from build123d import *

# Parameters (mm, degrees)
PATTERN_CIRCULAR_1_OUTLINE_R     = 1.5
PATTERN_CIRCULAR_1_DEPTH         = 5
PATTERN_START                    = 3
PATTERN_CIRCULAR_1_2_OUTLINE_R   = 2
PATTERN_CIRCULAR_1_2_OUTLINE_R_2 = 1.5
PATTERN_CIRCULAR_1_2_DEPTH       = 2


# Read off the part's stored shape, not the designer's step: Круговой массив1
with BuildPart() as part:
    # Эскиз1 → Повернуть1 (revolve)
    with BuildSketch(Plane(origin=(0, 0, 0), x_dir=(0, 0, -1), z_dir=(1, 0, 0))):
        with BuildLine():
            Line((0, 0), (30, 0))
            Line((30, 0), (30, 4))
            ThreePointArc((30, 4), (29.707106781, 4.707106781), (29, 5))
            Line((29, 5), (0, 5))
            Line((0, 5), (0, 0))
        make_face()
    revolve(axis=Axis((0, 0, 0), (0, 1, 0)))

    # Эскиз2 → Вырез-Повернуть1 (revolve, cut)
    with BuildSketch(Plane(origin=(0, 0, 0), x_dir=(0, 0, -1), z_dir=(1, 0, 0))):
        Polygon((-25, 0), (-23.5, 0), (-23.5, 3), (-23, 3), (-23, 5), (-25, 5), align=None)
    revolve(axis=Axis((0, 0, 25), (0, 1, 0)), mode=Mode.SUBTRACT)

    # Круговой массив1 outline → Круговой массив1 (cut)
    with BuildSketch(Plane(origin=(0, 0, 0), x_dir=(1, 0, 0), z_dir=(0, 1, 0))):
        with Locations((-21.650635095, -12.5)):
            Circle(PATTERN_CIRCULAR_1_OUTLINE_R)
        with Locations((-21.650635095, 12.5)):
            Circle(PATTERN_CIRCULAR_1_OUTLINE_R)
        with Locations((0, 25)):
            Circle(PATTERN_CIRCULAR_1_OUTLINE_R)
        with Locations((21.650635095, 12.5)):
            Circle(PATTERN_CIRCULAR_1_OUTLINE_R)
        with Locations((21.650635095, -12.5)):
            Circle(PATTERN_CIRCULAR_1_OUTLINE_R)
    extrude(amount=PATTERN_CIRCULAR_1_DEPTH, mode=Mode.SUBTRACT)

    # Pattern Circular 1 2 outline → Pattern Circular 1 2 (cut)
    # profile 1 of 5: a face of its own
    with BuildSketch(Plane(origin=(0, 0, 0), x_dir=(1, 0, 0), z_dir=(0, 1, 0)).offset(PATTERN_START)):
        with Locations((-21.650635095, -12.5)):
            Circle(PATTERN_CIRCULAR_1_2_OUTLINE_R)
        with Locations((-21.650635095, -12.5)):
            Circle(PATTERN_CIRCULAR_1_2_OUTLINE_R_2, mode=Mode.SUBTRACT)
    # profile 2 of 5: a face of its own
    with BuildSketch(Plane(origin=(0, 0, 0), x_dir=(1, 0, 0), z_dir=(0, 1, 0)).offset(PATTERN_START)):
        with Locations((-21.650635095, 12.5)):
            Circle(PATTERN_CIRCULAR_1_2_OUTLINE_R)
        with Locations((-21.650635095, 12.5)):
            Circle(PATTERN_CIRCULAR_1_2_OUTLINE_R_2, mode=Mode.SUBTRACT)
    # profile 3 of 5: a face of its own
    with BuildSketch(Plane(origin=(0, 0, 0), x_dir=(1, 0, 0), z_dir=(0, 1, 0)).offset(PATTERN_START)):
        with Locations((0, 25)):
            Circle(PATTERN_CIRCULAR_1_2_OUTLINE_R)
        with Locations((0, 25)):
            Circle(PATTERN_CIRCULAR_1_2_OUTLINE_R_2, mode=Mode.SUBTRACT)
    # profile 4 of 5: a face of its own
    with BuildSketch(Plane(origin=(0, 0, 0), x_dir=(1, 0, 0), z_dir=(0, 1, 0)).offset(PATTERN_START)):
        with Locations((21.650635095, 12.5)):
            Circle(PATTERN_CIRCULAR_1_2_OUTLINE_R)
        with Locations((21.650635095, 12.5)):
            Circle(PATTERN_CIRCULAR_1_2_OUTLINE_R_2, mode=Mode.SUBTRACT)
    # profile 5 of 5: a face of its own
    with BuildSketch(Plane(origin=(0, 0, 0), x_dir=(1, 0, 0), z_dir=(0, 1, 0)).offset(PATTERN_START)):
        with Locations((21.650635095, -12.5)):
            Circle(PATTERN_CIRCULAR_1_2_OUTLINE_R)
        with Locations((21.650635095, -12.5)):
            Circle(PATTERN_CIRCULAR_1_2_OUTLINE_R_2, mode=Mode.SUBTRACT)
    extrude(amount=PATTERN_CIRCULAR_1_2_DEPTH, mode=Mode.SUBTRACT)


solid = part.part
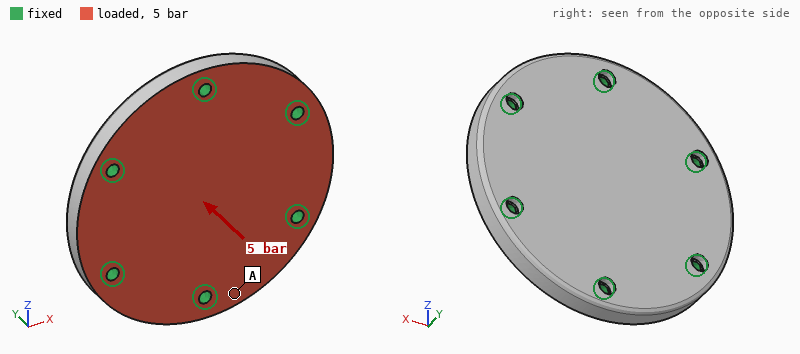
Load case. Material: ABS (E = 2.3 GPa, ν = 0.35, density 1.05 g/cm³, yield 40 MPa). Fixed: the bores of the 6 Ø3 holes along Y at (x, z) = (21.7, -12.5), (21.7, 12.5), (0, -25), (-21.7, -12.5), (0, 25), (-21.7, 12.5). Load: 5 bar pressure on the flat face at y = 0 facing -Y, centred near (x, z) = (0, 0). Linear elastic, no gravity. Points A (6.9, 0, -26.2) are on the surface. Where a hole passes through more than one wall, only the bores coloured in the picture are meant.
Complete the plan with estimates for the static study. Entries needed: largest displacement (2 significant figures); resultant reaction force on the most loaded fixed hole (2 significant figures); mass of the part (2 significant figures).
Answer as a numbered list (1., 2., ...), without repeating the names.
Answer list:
1. 0.23 mm
2. 240 N
3. 15 g
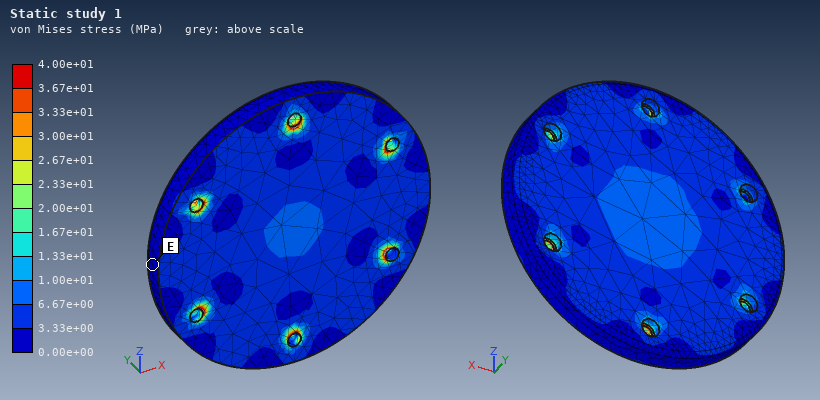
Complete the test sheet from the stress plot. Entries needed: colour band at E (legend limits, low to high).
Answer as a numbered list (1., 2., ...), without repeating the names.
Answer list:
1. 0.00e+00 to 3.33e+00 MPa
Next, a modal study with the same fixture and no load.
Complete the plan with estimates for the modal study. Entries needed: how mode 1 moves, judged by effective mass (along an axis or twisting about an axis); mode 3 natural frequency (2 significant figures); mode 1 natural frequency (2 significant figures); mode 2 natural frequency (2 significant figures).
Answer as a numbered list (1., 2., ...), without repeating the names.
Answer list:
1. along Y
2. 7200 Hz
3. 3900 Hz
4. 6900 Hz
